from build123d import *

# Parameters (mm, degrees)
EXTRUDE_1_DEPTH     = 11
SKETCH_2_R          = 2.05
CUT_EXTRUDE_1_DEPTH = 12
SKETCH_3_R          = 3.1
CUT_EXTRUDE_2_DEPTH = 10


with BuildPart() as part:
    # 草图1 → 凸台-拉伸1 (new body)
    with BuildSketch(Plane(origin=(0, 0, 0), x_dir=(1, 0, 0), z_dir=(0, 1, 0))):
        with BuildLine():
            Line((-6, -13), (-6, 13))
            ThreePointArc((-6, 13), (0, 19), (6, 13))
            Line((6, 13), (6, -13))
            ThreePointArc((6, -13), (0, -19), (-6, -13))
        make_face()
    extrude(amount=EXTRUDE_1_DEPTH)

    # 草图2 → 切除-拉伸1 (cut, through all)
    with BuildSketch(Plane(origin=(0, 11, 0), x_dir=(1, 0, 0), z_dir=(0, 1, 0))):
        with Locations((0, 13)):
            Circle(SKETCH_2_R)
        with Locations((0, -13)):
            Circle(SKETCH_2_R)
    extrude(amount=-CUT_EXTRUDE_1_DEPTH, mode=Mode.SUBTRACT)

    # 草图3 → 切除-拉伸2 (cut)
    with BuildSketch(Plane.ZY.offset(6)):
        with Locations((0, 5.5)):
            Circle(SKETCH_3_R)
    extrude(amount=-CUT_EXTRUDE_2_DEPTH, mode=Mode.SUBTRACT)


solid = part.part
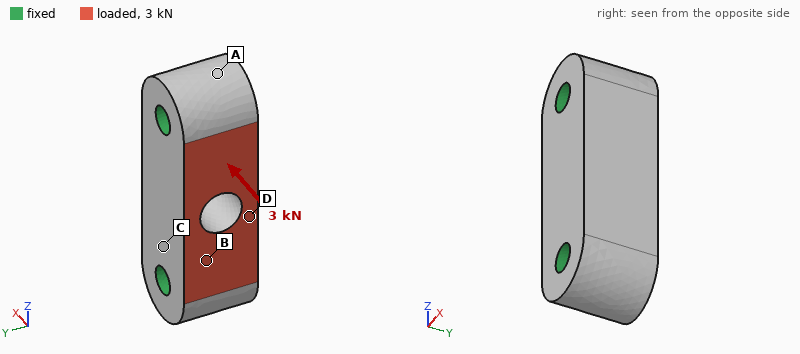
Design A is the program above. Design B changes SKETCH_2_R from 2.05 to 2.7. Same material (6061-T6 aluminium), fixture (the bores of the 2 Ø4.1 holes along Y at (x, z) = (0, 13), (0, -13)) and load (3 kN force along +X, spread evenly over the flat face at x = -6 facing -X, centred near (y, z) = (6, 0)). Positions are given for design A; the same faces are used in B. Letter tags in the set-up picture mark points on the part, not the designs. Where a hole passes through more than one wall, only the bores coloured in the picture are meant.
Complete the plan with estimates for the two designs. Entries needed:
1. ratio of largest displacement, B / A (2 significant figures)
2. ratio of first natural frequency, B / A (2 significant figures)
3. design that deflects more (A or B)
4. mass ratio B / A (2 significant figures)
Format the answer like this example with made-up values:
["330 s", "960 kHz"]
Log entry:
["0.81", "1.2", "A", "0.95"]
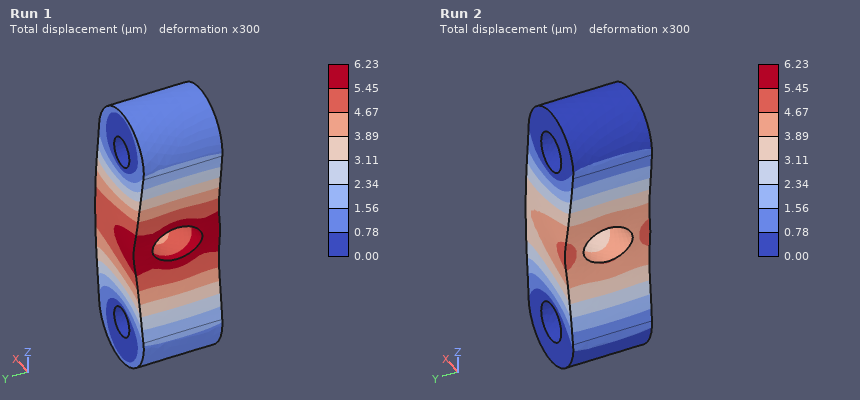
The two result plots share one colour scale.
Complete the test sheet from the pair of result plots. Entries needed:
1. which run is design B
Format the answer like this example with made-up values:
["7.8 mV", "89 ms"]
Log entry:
["Run 2"]
